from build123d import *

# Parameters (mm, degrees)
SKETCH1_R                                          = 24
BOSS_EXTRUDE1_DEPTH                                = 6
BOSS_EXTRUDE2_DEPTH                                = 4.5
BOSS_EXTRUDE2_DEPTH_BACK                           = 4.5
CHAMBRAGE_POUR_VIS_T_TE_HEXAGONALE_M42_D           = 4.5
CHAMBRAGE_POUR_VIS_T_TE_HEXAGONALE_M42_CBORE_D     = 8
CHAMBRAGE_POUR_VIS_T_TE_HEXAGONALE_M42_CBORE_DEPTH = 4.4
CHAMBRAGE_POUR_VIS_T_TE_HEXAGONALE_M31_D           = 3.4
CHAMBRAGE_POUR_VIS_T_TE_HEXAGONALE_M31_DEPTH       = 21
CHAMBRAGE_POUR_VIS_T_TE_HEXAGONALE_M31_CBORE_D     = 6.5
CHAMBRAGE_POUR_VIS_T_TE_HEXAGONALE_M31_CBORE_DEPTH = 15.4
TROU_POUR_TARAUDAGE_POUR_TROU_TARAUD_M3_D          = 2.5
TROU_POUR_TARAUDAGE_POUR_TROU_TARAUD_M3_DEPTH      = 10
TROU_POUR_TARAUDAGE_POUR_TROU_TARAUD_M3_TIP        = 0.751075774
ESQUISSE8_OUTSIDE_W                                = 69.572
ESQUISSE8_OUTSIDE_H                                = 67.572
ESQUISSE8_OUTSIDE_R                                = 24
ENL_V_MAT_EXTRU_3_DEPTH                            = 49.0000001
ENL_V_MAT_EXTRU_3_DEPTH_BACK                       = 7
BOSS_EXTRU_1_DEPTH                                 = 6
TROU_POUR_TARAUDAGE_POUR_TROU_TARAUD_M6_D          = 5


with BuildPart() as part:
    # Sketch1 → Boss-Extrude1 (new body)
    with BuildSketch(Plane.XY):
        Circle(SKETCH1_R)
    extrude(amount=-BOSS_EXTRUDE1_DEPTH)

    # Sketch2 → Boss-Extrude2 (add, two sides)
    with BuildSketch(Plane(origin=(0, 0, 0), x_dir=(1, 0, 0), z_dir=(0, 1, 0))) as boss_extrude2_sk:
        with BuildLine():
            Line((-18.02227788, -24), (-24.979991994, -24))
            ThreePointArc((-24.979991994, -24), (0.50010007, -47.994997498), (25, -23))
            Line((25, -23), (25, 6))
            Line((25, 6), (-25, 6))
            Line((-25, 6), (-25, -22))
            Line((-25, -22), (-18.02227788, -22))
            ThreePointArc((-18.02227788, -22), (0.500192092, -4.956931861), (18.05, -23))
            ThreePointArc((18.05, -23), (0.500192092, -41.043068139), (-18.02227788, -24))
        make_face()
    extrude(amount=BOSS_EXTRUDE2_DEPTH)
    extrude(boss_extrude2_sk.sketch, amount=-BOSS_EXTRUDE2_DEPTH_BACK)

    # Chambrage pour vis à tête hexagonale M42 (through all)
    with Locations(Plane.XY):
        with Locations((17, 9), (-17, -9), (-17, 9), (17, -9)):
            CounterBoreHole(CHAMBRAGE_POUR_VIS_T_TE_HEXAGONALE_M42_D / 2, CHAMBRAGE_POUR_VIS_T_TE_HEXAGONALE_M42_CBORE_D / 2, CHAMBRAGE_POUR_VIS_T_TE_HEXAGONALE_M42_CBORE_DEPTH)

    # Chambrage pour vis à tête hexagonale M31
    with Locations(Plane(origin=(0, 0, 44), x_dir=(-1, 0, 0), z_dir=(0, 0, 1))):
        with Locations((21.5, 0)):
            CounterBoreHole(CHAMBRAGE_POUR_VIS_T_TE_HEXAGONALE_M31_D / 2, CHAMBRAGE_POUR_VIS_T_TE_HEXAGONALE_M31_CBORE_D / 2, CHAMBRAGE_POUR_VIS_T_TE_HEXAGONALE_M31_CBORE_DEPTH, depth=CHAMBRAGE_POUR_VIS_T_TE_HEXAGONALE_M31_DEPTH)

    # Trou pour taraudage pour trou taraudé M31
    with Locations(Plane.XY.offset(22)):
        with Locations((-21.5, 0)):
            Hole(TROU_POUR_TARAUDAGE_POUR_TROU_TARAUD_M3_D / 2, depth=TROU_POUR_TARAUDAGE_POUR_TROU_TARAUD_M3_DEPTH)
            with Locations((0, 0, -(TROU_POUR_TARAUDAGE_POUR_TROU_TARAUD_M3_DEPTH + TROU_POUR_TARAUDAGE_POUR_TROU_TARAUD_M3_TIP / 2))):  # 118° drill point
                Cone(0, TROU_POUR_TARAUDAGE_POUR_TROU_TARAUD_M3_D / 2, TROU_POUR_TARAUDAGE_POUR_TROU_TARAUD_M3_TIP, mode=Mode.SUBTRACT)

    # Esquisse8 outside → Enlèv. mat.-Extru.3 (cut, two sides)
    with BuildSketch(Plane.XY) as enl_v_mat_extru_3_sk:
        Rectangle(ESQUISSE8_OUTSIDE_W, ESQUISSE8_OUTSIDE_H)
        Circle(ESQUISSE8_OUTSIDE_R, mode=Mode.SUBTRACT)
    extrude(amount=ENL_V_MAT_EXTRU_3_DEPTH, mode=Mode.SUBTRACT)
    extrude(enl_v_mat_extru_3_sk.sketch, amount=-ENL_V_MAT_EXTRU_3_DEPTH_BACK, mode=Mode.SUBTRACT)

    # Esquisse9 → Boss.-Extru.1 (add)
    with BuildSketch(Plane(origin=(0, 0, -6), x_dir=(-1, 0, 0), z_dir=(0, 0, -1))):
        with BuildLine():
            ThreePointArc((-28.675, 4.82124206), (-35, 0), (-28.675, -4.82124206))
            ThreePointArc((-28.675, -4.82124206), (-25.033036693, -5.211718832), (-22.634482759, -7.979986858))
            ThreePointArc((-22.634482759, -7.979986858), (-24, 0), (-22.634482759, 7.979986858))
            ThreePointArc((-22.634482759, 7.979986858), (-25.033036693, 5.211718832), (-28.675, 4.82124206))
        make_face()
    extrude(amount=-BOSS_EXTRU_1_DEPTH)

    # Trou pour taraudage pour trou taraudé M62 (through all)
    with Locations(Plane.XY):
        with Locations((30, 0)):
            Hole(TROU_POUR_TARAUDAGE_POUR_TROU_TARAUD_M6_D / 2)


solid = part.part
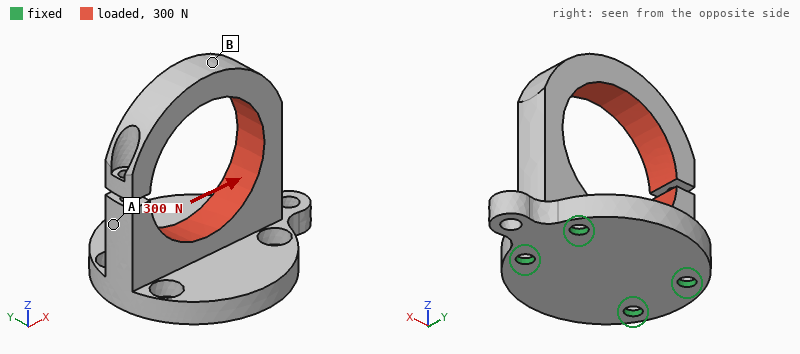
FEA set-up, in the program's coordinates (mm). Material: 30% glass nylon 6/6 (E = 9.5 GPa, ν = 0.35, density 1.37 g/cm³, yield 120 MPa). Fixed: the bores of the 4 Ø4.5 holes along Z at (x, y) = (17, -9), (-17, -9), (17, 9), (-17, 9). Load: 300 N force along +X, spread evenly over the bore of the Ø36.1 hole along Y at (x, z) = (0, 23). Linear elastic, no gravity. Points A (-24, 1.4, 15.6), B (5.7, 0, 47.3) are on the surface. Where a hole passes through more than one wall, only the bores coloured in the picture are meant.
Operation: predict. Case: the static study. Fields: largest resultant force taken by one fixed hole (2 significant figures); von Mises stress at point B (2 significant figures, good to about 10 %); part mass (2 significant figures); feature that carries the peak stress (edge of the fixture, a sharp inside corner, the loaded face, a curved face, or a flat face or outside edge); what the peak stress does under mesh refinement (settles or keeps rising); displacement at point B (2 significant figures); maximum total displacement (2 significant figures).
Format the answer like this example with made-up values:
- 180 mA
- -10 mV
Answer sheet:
- 210 N
- 7.4 MPa
- 27 g
- edge of the fixture
- keeps rising
- 0.87 mm
- 1.1 mm
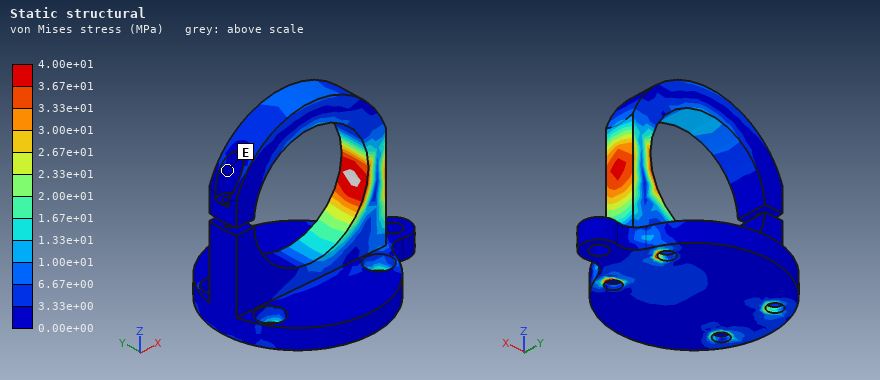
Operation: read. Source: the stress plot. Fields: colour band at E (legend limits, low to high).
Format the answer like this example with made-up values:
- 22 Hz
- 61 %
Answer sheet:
- 0.00e+00 to 3.33e+00 MPa
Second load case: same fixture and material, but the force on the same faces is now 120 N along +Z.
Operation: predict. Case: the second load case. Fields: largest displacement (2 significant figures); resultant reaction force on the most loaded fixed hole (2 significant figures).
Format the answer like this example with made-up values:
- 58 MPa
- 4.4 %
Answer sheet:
- 0.94 mm
- 41 N
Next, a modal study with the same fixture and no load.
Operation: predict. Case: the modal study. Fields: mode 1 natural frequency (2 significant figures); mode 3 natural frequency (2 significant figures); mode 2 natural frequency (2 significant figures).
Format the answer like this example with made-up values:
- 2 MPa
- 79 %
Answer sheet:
- 590 Hz
- 1600 Hz
- 610 Hz
